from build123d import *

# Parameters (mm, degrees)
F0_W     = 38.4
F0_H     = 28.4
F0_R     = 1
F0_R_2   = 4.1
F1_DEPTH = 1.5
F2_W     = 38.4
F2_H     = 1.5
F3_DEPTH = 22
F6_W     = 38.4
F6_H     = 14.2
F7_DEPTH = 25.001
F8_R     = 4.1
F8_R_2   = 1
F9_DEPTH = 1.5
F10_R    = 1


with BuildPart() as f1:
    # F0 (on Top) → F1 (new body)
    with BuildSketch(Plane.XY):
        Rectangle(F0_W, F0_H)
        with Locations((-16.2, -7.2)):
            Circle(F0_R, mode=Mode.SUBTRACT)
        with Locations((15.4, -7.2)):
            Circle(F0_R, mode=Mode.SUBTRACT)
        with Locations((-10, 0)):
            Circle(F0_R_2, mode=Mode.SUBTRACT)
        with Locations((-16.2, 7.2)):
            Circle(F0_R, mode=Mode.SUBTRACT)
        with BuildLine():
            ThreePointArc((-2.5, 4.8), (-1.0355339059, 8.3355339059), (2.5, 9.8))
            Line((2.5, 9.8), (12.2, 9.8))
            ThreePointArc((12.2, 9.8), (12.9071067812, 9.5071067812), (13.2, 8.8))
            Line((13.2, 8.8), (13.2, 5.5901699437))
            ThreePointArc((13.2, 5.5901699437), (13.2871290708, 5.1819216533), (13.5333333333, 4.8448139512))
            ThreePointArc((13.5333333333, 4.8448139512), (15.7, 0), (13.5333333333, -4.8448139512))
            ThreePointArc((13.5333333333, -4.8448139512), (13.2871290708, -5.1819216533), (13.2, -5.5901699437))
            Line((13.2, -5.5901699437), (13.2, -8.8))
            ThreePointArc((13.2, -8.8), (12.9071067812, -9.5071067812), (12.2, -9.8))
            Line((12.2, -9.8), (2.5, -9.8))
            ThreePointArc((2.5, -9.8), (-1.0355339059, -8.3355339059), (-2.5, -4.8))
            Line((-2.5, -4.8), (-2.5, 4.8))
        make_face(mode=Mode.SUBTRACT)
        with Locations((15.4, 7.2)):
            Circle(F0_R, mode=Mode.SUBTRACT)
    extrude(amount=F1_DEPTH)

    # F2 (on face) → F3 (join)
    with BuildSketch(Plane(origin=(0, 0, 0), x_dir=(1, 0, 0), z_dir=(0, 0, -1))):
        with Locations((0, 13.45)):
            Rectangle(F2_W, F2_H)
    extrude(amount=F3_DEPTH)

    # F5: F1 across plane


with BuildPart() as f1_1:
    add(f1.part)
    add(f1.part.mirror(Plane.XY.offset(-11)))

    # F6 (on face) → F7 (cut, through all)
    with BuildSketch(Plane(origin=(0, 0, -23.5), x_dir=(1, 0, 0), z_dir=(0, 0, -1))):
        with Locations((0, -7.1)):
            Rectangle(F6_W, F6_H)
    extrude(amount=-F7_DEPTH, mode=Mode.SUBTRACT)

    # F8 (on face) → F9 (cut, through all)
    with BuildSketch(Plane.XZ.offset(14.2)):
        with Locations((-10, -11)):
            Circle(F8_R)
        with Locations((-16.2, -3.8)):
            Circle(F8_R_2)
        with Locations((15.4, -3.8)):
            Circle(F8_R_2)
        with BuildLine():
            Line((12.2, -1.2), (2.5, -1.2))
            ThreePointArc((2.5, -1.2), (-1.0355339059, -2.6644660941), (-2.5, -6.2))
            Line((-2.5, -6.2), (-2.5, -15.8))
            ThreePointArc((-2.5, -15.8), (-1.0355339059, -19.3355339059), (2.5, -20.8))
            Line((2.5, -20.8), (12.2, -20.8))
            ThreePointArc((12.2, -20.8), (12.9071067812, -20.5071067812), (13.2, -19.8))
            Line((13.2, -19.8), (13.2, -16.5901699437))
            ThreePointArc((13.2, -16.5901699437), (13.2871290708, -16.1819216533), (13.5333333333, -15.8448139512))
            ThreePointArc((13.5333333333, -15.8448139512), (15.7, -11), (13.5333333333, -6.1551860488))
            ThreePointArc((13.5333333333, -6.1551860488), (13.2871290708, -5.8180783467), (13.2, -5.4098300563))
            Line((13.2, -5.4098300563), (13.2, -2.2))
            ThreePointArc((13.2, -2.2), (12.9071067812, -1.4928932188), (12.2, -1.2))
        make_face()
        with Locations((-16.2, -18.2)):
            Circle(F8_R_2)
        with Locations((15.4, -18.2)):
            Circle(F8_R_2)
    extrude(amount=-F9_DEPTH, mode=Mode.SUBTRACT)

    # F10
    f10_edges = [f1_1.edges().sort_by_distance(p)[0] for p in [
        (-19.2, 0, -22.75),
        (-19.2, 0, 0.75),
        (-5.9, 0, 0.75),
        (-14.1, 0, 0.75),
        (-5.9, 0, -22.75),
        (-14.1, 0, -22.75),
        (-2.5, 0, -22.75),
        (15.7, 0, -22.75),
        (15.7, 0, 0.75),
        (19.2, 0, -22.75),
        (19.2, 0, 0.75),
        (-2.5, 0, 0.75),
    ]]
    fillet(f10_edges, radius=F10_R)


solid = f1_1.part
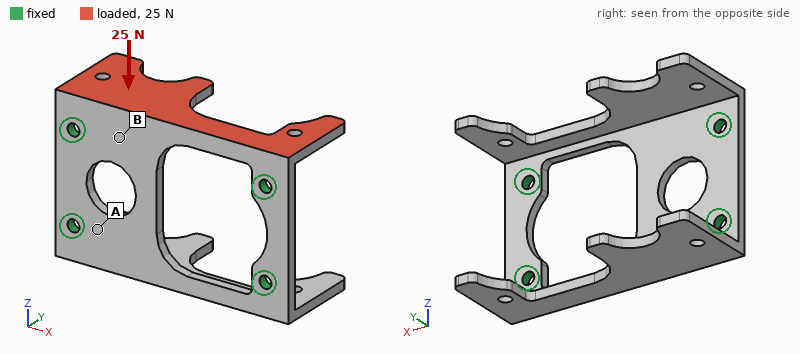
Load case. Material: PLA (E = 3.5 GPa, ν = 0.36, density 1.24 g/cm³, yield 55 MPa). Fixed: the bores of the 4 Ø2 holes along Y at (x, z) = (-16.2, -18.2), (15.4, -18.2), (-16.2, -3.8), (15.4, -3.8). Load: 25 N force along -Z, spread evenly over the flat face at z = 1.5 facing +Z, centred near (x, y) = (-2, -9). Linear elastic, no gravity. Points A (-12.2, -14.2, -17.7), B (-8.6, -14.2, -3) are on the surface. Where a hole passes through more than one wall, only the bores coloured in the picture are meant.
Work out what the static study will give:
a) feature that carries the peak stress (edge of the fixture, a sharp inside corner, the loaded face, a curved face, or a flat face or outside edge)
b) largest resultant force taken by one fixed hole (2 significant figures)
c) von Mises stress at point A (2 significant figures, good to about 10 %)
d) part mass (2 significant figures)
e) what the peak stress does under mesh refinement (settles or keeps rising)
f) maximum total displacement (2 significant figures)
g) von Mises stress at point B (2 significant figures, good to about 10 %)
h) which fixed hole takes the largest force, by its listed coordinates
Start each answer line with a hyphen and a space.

- edge of the fixture
- 13 N
- 2.4 MPa
- 2.2 g
- keeps rising
- 0.52 mm
- 6.7 MPa
- (-16.2, -3.8)
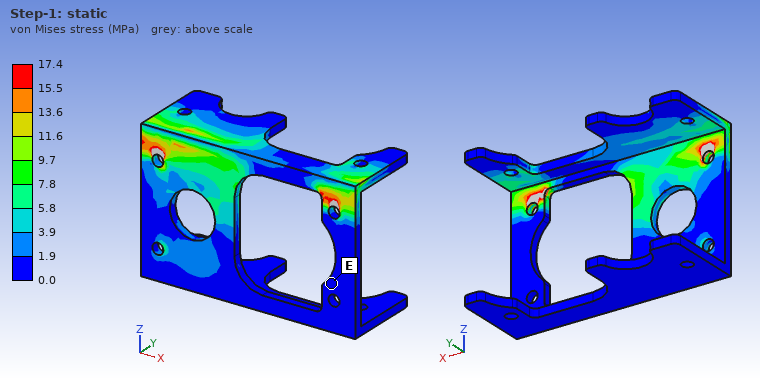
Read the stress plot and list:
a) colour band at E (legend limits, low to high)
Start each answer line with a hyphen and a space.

- 0.0 to 1.9 MPa
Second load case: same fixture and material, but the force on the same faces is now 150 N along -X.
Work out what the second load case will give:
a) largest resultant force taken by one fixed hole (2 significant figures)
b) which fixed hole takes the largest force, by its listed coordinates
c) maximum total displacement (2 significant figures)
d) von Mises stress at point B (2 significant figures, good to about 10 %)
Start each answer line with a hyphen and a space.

- 110 N
- (-16.2, -3.8)
- 0.31 mm
- 5.2 MPa
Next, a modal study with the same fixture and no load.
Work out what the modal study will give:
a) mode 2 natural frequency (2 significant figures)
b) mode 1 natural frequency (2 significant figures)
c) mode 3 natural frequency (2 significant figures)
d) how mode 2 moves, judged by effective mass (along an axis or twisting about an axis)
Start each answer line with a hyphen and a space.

- 1800 Hz
- 1700 Hz
- 2100 Hz
- along Z
